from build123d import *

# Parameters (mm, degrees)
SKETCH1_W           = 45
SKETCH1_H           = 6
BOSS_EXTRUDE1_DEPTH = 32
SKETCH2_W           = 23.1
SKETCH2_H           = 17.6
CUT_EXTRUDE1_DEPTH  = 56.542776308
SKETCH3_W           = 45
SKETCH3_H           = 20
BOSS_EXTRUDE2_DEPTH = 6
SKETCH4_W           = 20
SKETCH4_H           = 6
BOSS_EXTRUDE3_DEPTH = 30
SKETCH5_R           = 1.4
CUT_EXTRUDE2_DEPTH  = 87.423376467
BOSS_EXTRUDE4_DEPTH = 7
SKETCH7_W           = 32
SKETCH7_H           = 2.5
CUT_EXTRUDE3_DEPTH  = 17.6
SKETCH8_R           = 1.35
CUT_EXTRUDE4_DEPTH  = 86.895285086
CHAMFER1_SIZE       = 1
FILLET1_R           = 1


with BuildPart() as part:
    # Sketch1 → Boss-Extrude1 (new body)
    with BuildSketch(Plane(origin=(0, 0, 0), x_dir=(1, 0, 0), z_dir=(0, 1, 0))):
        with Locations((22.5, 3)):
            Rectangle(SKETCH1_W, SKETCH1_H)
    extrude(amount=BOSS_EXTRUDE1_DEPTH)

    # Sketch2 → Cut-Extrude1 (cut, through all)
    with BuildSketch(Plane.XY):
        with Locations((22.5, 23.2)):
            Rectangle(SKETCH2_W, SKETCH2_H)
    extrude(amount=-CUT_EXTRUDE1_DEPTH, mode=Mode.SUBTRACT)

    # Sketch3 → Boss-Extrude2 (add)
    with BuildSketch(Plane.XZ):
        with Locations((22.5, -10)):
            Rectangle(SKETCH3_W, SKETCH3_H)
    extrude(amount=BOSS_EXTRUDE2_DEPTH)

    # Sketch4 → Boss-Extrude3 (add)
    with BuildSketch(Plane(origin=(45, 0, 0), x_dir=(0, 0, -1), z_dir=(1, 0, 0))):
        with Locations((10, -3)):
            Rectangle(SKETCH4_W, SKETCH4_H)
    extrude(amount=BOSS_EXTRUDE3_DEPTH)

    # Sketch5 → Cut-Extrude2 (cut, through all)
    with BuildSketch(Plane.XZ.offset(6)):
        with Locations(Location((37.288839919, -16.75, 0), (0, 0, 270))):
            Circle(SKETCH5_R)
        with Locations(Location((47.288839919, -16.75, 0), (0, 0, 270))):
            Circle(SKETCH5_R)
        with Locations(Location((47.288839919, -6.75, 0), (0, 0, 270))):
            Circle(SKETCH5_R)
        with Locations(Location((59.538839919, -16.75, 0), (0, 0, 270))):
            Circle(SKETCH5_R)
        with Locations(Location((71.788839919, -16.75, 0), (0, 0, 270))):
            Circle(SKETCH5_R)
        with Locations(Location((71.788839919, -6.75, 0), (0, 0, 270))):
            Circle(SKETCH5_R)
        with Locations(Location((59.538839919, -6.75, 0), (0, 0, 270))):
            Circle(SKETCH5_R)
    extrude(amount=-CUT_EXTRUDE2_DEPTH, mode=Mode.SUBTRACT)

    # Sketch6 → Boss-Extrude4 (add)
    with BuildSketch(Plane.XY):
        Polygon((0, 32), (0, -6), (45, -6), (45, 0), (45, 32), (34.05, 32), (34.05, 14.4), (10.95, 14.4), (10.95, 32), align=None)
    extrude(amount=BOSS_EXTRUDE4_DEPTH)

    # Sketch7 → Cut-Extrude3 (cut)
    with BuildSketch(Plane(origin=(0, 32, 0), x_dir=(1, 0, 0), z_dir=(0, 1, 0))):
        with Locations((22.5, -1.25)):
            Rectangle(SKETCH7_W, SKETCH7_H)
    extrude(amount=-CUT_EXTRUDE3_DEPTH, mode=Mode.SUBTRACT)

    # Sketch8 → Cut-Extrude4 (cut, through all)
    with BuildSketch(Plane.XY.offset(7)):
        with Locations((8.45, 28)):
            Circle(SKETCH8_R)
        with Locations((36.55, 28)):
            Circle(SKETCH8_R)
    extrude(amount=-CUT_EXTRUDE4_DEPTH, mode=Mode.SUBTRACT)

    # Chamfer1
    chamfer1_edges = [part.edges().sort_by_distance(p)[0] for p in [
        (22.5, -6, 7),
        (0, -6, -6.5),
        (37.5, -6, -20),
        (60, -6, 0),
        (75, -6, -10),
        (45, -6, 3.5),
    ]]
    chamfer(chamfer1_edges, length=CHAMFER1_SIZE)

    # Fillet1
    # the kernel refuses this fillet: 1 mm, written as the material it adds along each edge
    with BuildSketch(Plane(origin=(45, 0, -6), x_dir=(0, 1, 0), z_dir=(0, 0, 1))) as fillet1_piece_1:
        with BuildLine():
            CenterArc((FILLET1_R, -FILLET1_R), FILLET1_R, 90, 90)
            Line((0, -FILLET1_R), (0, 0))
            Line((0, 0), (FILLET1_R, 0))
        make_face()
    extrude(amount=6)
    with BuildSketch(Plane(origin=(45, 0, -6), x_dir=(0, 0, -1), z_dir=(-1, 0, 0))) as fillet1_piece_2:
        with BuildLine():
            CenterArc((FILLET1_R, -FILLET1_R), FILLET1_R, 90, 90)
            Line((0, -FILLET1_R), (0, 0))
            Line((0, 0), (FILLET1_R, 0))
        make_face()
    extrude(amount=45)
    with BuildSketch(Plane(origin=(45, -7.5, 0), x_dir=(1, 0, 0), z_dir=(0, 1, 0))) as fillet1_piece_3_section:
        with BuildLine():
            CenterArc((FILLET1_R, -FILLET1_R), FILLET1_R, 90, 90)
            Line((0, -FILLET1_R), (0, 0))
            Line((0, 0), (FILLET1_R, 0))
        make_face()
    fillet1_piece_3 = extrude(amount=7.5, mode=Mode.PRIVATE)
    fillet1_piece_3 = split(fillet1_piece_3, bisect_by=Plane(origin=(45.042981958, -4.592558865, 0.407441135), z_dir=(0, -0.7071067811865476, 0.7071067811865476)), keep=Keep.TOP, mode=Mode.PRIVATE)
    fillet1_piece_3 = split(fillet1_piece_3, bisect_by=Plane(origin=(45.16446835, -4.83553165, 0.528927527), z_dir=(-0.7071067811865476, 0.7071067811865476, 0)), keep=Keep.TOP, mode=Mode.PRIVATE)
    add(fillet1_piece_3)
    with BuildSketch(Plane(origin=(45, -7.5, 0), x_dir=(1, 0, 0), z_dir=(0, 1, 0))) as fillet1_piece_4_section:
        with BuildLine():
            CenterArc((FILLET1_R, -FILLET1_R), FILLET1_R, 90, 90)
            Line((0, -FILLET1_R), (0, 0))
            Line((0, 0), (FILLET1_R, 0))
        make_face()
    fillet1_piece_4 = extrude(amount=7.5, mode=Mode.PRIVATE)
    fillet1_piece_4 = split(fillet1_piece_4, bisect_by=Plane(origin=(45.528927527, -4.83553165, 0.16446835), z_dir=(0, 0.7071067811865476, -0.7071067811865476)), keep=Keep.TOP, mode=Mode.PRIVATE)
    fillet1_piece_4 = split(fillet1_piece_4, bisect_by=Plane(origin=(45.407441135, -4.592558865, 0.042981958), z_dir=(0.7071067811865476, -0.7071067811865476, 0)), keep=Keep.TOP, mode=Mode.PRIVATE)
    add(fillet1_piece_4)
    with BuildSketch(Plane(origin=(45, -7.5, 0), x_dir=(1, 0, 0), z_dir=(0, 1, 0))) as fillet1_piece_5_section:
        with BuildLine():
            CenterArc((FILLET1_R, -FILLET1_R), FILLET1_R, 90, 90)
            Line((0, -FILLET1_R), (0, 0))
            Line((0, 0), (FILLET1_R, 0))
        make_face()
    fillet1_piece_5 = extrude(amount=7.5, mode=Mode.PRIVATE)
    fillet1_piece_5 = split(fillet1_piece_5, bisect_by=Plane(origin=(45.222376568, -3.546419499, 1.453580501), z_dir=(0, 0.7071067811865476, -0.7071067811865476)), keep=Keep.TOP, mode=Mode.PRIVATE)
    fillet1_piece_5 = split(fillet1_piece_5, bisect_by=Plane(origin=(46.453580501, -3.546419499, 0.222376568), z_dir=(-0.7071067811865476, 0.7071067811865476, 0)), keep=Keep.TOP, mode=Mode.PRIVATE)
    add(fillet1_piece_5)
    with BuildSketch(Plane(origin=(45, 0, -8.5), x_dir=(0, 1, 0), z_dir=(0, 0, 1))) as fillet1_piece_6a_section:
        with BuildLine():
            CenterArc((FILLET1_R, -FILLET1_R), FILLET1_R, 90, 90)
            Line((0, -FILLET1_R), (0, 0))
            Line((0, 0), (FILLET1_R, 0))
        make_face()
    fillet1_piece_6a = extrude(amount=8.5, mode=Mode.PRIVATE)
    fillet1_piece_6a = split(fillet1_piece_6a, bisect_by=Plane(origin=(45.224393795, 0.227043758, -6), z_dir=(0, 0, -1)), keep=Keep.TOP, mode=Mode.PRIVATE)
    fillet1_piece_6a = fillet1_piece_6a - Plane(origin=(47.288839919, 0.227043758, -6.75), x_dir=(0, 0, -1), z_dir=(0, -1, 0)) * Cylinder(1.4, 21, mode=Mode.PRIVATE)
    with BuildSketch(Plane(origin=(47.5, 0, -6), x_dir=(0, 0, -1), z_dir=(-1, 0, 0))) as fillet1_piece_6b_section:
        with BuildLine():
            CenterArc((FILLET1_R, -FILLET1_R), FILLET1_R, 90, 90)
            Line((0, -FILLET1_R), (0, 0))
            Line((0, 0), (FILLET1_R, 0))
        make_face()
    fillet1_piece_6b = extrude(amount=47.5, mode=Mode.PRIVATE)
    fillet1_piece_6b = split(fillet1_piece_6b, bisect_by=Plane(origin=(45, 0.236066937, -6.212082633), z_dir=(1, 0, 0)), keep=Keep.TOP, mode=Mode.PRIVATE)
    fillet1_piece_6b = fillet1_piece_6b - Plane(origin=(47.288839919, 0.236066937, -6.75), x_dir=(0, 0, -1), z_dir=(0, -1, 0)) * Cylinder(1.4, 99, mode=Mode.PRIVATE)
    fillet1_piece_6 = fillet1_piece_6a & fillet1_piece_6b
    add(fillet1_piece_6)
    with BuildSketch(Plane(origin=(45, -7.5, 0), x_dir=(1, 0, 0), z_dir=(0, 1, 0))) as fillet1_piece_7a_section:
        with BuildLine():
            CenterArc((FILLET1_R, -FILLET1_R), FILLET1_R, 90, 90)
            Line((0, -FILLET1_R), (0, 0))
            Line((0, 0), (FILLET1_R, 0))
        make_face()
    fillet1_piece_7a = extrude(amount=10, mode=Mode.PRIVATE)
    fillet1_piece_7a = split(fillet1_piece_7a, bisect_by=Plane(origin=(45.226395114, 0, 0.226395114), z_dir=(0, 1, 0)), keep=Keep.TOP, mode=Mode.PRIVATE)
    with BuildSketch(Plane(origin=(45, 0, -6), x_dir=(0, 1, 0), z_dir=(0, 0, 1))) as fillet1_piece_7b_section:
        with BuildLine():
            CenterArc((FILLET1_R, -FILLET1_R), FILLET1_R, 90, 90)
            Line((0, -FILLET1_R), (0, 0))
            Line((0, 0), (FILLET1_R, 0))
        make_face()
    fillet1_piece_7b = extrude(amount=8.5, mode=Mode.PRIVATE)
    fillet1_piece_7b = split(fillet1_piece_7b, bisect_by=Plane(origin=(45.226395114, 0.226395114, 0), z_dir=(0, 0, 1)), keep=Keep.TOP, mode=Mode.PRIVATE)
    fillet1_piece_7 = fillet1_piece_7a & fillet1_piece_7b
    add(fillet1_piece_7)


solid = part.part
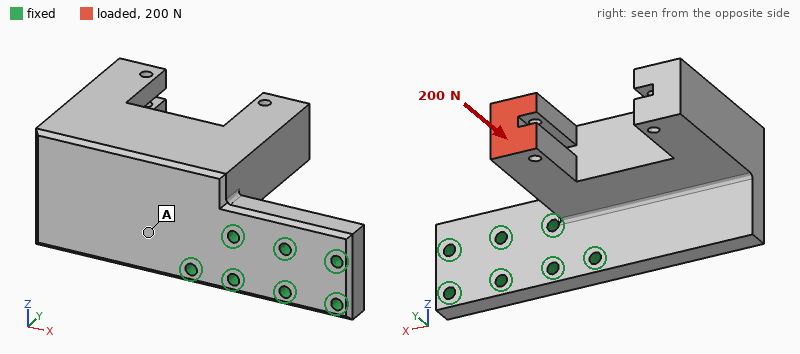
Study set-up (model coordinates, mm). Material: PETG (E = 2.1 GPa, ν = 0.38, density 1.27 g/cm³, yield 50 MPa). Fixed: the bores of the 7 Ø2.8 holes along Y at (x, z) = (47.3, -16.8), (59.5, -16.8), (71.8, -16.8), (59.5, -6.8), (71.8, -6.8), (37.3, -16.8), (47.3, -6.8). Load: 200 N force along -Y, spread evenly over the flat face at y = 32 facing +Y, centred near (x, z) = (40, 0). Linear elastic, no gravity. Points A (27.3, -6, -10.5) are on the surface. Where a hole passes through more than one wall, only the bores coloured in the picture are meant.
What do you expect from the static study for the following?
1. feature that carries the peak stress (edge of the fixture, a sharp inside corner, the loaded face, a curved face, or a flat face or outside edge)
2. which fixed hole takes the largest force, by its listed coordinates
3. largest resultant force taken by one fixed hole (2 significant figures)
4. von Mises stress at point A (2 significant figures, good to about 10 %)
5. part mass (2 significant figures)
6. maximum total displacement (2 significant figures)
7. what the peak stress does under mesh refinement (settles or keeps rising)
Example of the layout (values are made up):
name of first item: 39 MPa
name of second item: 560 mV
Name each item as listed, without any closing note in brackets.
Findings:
feature that carries the peak stress: edge of the fixture
which fixed hole takes the largest force, by its listed coordinates: (47.3, -6.8)
largest resultant force taken by one fixed hole: 210 N
von Mises stress at point A: 2.4 MPa
part mass: 30 g
maximum total displacement: 0.62 mm
what the peak stress does under mesh refinement: keeps rising
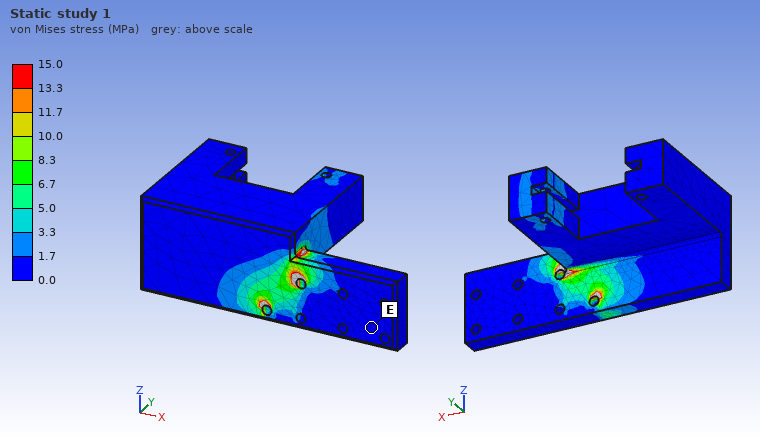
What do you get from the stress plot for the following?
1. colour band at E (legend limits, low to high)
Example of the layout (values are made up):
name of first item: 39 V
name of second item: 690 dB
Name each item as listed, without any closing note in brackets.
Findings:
colour band at E: 0.0 to 1.7 MPa
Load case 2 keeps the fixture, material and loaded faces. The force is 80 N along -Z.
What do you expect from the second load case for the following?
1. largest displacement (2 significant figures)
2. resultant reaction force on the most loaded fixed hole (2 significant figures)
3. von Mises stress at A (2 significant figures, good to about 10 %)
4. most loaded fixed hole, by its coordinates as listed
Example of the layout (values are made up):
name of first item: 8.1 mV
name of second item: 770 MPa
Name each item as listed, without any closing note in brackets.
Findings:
largest displacement: 1.0 mm
resultant reaction force on the most loaded fixed hole: 140 N
von Mises stress at A: 6.4 MPa
most loaded fixed hole, by its coordinates as listed: (47.3, -6.8)
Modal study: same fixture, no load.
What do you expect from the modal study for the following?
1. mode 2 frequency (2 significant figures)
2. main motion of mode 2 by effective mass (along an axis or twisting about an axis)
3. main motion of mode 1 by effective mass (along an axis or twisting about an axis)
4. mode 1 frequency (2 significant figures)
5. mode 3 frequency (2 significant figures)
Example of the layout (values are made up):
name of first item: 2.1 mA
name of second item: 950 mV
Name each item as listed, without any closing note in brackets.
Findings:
mode 2 frequency: 820 Hz
main motion of mode 2 by effective mass: along Z
main motion of mode 1 by effective mass: along Y
mode 1 frequency: 420 Hz
mode 3 frequency: 1400 Hz
